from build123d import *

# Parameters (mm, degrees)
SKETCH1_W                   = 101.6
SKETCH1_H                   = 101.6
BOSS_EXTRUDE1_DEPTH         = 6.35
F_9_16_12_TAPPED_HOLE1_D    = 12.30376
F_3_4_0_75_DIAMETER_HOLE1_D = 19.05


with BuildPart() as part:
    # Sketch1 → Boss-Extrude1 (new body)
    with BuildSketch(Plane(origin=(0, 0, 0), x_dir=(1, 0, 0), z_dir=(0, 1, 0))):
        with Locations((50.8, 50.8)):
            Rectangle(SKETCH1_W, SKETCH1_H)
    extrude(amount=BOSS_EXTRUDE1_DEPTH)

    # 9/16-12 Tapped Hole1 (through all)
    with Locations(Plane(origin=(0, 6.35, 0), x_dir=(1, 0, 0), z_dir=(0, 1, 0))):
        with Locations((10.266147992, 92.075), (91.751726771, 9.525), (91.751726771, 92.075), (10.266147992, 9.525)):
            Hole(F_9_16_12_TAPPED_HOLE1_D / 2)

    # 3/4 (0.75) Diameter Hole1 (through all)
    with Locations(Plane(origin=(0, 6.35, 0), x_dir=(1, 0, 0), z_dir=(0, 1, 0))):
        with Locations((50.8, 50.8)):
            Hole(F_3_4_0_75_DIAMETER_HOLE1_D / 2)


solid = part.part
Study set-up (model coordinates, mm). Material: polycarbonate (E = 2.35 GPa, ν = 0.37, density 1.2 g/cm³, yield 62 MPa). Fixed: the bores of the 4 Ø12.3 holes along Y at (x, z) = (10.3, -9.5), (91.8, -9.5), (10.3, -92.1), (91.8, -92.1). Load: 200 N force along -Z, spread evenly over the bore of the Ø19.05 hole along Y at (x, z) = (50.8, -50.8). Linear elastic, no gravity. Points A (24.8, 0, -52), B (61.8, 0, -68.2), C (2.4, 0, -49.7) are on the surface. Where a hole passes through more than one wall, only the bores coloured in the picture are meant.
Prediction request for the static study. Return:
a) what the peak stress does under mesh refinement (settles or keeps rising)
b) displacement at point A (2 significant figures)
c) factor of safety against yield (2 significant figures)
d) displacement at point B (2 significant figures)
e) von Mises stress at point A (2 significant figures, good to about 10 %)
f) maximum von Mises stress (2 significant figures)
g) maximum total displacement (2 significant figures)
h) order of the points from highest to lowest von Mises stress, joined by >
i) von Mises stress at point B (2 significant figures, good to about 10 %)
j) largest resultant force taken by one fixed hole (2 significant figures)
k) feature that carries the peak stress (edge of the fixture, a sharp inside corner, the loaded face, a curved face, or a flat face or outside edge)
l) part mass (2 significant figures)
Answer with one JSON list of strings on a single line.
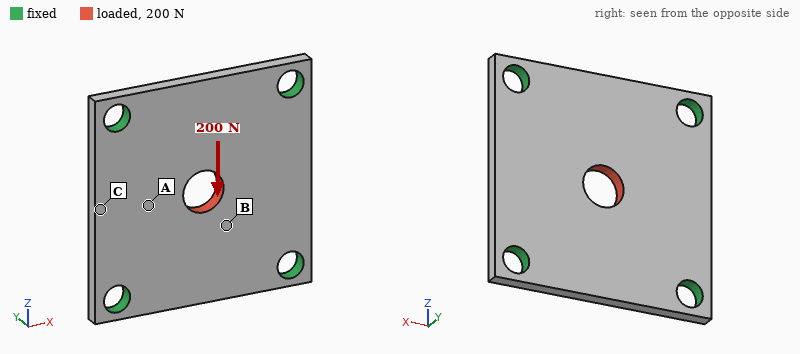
["settles", "3.9 µm", "68", "6.8 µm", "0.23 MPa", "0.92 MPa", "9.6 µm", "B > A > C", "0.37 MPa", "57 N", "the loaded face", "73 g"]
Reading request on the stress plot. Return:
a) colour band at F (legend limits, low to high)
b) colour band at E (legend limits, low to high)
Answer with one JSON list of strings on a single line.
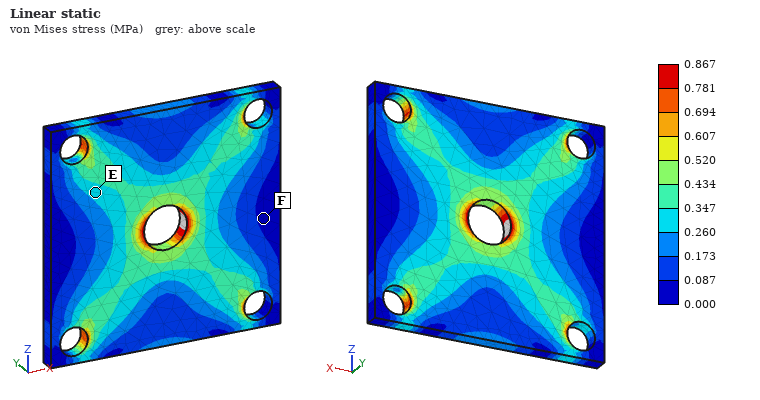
["0.000 to 0.087 MPa", "0.260 to 0.347 MPa"]
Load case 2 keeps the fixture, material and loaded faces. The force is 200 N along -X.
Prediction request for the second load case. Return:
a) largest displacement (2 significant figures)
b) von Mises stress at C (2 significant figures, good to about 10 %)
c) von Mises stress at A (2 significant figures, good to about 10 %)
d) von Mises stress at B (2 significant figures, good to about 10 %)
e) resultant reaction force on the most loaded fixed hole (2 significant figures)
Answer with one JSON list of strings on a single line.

["9.8 µm", "0.19 MPa", "0.20 MPa", "0.35 MPa", "57 N"]
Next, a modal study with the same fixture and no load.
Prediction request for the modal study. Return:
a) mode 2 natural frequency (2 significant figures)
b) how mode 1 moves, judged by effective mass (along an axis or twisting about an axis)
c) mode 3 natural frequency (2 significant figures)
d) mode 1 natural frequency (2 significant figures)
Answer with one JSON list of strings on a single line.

["1700 Hz", "along Y", "1800 Hz", "1100 Hz"]
